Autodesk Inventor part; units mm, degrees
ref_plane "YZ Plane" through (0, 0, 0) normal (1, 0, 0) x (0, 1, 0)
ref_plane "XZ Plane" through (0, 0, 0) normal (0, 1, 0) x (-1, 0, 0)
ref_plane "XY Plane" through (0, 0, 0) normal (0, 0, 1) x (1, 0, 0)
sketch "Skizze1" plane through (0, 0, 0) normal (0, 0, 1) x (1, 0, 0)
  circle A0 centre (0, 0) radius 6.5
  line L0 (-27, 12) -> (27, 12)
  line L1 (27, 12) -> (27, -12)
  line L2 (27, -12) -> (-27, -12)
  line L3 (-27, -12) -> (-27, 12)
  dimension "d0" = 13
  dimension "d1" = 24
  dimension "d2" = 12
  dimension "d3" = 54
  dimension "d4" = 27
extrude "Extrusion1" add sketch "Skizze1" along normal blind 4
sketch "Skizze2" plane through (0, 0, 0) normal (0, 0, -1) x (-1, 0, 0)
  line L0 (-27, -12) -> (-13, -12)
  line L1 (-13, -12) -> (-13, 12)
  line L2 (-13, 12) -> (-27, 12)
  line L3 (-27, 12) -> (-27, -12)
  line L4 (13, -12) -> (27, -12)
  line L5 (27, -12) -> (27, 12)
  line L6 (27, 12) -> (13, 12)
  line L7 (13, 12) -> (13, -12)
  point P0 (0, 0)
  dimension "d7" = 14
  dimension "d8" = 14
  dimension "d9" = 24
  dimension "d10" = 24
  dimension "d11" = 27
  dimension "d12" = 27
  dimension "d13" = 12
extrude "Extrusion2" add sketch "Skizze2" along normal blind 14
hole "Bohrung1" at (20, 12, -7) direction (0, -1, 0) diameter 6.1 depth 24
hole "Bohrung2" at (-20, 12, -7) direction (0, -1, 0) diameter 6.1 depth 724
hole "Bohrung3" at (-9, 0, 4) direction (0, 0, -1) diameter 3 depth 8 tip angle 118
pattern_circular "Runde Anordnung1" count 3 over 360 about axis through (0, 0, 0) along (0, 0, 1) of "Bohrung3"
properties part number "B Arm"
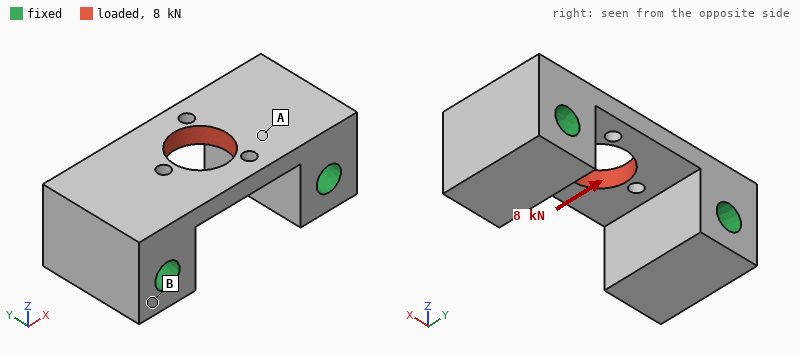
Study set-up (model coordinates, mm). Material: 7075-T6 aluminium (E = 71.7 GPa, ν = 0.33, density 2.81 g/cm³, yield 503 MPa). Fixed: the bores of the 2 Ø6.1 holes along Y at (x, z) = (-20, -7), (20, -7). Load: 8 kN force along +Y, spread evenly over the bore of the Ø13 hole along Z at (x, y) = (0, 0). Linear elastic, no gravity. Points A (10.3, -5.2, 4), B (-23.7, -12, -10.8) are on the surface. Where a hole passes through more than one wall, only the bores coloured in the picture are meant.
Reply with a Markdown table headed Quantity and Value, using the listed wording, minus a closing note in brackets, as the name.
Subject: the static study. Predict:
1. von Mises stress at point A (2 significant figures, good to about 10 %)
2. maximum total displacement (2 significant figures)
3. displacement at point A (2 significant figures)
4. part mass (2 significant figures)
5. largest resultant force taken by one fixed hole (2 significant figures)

| Quantity | Value |
|---|---|
| von Mises stress at point A | 69 MPa |
| maximum total displacement | 45 µm |
| displacement at point A | 18 µm |
| part mass | 35 g |
| largest resultant force taken by one fixed hole | 4.0 kN |
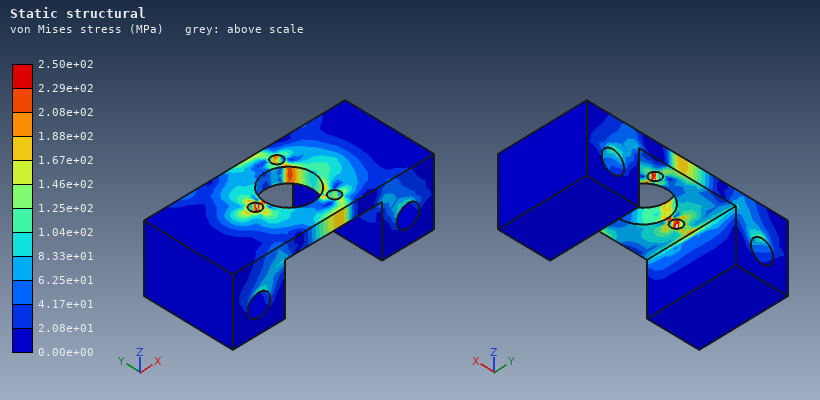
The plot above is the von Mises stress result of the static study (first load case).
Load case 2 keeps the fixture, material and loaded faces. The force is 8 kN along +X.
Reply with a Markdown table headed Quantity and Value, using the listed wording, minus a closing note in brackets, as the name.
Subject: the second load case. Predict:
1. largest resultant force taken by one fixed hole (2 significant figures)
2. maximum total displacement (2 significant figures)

| Quantity | Value |
|---|---|
| largest resultant force taken by one fixed hole | 4.2 kN |
| maximum total displacement | 21 µm |
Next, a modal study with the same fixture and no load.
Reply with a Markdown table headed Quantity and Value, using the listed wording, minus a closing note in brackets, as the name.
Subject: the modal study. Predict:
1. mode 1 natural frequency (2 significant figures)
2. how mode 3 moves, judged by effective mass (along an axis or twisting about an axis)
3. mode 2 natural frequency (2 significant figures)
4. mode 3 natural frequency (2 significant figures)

| Quantity | Value |
|---|---|
| mode 1 natural frequency | 23 kHz |
| how mode 3 moves, judged by effective mass | along X |
| mode 2 natural frequency | 25 kHz |
| mode 3 natural frequency | 36 kHz |
